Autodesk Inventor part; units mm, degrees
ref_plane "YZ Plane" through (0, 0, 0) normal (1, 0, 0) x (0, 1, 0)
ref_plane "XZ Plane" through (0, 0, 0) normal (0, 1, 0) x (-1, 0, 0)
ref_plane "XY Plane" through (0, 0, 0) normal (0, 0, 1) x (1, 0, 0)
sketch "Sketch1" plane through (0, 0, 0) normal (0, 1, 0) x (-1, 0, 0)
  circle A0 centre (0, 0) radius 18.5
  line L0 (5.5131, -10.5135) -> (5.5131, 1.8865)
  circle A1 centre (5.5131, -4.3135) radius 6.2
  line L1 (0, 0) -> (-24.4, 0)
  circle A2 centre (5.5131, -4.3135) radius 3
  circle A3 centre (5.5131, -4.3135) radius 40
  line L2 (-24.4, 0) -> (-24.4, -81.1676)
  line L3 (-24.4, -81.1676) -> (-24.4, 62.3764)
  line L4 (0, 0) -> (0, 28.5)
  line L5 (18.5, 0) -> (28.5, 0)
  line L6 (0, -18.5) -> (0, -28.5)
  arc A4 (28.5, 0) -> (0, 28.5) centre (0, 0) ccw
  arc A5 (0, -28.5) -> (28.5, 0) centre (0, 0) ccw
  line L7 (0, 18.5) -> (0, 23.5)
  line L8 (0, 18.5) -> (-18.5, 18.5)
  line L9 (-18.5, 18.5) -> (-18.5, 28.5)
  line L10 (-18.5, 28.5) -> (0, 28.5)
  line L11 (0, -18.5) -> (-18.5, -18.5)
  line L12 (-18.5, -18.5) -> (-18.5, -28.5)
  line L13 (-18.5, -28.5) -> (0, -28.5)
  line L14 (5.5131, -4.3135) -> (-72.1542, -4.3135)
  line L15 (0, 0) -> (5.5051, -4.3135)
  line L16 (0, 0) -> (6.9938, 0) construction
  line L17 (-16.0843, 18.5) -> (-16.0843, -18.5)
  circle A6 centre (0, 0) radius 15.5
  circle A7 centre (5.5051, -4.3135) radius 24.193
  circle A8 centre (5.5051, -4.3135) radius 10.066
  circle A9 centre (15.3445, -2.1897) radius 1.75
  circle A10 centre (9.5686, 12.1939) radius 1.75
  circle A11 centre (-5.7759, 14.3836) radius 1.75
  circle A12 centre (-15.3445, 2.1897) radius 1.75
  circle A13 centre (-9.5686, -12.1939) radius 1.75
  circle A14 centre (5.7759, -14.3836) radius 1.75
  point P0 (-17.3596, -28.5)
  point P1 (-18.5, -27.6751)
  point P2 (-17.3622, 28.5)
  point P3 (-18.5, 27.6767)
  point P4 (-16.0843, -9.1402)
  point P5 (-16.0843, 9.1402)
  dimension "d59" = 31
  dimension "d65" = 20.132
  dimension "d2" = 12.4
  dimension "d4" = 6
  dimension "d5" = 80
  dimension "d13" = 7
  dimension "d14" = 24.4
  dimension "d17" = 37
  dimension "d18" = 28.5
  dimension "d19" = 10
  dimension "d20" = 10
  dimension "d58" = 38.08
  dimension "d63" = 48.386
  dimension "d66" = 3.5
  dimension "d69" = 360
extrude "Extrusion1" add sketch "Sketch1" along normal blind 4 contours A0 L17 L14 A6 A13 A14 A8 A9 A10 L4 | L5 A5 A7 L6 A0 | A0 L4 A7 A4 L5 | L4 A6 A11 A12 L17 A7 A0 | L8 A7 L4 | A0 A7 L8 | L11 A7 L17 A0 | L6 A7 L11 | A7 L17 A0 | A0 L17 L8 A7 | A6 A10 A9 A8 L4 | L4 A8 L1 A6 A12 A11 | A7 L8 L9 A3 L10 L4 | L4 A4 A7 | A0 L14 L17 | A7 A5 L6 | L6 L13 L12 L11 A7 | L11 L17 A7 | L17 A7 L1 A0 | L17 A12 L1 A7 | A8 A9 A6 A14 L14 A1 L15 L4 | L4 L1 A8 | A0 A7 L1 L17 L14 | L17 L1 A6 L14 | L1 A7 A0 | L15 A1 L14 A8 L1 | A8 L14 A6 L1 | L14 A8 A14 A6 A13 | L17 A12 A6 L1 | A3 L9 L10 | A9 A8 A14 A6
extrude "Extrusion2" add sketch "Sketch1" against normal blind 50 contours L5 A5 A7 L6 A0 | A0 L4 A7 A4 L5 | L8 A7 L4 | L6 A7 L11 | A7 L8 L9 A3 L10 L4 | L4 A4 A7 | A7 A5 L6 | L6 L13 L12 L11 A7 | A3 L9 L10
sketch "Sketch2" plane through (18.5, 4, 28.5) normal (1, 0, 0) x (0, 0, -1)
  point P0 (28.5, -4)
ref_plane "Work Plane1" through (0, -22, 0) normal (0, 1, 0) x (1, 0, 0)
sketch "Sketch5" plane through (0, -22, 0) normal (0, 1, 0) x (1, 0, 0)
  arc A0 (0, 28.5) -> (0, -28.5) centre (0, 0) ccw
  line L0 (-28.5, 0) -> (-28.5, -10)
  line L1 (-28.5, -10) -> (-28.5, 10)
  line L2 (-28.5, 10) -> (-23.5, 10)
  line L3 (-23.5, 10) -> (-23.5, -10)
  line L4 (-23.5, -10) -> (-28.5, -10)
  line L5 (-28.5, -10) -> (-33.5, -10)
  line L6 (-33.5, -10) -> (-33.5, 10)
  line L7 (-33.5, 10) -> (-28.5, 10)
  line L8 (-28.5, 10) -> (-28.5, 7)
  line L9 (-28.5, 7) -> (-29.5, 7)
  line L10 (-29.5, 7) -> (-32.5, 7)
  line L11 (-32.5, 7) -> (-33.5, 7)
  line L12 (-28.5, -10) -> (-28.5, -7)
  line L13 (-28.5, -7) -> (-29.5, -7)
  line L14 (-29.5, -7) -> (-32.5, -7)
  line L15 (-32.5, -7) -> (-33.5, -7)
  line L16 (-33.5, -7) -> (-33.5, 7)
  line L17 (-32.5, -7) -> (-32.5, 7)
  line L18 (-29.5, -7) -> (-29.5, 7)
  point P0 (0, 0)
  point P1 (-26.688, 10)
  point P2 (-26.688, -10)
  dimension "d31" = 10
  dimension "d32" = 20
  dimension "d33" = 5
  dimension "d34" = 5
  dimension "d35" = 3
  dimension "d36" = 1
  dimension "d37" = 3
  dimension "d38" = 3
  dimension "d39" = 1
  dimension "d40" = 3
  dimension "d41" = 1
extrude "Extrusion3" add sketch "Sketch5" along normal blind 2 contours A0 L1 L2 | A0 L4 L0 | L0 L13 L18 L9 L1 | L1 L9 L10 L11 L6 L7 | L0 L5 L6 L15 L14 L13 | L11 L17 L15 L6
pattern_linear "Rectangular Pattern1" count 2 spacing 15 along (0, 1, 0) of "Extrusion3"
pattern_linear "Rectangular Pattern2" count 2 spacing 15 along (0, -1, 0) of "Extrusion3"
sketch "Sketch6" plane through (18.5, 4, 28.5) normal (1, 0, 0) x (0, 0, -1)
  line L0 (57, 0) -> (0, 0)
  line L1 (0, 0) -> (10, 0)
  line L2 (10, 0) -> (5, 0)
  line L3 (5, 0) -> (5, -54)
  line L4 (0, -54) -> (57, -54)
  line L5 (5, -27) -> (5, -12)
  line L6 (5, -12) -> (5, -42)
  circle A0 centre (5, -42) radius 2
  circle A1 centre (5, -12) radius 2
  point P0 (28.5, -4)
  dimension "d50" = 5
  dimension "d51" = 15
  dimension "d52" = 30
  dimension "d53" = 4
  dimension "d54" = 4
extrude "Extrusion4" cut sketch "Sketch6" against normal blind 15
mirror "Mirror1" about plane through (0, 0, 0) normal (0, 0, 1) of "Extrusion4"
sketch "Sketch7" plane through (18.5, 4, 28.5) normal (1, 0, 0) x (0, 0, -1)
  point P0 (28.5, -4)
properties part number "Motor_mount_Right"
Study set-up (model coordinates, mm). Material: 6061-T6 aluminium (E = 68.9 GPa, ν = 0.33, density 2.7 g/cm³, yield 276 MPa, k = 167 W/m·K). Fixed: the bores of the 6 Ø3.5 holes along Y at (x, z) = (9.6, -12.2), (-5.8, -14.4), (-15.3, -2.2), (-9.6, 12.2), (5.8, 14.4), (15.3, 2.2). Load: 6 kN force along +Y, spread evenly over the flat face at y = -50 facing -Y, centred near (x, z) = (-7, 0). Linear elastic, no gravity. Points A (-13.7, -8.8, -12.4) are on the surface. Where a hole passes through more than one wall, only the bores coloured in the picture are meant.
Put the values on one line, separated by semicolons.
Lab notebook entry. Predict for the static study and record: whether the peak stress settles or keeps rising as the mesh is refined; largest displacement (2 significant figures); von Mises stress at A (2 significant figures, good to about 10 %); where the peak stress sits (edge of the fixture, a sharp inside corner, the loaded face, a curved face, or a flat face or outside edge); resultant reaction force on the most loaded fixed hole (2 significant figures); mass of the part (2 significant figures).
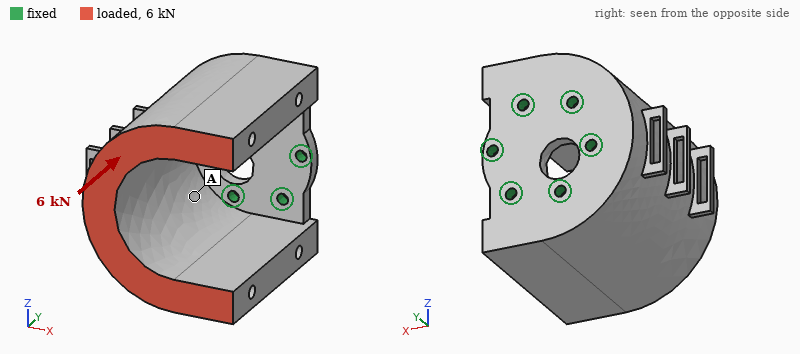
keeps rising; 20 µm; 15 MPa; edge of the fixture; 1.6 kN; 170 g
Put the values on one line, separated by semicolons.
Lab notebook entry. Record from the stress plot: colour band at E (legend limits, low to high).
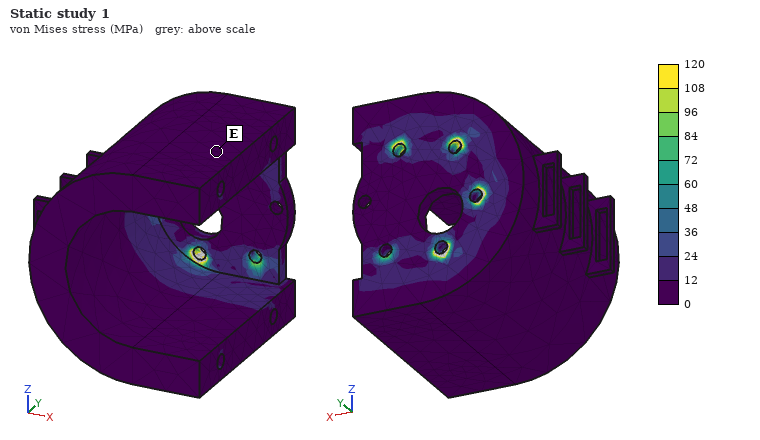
0 to 12 MPa
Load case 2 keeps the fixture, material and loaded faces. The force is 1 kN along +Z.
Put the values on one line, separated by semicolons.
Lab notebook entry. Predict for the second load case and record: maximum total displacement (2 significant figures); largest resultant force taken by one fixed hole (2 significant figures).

0.12 mm; 1.6 kN
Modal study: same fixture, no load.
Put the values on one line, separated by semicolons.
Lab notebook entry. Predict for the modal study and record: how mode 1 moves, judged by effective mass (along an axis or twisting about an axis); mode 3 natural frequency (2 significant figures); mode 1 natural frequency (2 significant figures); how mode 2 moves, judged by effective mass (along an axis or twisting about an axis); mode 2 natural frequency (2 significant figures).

along Z; 5100 Hz; 2200 Hz; along X; 2800 Hz
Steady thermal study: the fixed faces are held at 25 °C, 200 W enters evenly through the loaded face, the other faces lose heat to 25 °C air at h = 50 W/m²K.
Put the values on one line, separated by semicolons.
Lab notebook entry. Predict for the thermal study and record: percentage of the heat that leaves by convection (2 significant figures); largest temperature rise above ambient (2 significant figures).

16 %; 72 K
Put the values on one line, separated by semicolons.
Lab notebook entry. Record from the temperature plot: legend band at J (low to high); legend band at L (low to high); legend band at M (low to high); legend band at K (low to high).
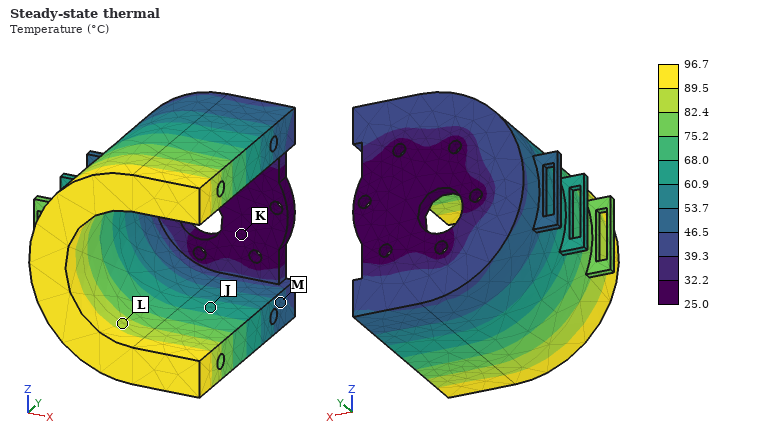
60.9 to 68.0 °C; 82.4 to 89.5 °C; 46.5 to 53.7 °C; 25.0 to 32.2 °C
